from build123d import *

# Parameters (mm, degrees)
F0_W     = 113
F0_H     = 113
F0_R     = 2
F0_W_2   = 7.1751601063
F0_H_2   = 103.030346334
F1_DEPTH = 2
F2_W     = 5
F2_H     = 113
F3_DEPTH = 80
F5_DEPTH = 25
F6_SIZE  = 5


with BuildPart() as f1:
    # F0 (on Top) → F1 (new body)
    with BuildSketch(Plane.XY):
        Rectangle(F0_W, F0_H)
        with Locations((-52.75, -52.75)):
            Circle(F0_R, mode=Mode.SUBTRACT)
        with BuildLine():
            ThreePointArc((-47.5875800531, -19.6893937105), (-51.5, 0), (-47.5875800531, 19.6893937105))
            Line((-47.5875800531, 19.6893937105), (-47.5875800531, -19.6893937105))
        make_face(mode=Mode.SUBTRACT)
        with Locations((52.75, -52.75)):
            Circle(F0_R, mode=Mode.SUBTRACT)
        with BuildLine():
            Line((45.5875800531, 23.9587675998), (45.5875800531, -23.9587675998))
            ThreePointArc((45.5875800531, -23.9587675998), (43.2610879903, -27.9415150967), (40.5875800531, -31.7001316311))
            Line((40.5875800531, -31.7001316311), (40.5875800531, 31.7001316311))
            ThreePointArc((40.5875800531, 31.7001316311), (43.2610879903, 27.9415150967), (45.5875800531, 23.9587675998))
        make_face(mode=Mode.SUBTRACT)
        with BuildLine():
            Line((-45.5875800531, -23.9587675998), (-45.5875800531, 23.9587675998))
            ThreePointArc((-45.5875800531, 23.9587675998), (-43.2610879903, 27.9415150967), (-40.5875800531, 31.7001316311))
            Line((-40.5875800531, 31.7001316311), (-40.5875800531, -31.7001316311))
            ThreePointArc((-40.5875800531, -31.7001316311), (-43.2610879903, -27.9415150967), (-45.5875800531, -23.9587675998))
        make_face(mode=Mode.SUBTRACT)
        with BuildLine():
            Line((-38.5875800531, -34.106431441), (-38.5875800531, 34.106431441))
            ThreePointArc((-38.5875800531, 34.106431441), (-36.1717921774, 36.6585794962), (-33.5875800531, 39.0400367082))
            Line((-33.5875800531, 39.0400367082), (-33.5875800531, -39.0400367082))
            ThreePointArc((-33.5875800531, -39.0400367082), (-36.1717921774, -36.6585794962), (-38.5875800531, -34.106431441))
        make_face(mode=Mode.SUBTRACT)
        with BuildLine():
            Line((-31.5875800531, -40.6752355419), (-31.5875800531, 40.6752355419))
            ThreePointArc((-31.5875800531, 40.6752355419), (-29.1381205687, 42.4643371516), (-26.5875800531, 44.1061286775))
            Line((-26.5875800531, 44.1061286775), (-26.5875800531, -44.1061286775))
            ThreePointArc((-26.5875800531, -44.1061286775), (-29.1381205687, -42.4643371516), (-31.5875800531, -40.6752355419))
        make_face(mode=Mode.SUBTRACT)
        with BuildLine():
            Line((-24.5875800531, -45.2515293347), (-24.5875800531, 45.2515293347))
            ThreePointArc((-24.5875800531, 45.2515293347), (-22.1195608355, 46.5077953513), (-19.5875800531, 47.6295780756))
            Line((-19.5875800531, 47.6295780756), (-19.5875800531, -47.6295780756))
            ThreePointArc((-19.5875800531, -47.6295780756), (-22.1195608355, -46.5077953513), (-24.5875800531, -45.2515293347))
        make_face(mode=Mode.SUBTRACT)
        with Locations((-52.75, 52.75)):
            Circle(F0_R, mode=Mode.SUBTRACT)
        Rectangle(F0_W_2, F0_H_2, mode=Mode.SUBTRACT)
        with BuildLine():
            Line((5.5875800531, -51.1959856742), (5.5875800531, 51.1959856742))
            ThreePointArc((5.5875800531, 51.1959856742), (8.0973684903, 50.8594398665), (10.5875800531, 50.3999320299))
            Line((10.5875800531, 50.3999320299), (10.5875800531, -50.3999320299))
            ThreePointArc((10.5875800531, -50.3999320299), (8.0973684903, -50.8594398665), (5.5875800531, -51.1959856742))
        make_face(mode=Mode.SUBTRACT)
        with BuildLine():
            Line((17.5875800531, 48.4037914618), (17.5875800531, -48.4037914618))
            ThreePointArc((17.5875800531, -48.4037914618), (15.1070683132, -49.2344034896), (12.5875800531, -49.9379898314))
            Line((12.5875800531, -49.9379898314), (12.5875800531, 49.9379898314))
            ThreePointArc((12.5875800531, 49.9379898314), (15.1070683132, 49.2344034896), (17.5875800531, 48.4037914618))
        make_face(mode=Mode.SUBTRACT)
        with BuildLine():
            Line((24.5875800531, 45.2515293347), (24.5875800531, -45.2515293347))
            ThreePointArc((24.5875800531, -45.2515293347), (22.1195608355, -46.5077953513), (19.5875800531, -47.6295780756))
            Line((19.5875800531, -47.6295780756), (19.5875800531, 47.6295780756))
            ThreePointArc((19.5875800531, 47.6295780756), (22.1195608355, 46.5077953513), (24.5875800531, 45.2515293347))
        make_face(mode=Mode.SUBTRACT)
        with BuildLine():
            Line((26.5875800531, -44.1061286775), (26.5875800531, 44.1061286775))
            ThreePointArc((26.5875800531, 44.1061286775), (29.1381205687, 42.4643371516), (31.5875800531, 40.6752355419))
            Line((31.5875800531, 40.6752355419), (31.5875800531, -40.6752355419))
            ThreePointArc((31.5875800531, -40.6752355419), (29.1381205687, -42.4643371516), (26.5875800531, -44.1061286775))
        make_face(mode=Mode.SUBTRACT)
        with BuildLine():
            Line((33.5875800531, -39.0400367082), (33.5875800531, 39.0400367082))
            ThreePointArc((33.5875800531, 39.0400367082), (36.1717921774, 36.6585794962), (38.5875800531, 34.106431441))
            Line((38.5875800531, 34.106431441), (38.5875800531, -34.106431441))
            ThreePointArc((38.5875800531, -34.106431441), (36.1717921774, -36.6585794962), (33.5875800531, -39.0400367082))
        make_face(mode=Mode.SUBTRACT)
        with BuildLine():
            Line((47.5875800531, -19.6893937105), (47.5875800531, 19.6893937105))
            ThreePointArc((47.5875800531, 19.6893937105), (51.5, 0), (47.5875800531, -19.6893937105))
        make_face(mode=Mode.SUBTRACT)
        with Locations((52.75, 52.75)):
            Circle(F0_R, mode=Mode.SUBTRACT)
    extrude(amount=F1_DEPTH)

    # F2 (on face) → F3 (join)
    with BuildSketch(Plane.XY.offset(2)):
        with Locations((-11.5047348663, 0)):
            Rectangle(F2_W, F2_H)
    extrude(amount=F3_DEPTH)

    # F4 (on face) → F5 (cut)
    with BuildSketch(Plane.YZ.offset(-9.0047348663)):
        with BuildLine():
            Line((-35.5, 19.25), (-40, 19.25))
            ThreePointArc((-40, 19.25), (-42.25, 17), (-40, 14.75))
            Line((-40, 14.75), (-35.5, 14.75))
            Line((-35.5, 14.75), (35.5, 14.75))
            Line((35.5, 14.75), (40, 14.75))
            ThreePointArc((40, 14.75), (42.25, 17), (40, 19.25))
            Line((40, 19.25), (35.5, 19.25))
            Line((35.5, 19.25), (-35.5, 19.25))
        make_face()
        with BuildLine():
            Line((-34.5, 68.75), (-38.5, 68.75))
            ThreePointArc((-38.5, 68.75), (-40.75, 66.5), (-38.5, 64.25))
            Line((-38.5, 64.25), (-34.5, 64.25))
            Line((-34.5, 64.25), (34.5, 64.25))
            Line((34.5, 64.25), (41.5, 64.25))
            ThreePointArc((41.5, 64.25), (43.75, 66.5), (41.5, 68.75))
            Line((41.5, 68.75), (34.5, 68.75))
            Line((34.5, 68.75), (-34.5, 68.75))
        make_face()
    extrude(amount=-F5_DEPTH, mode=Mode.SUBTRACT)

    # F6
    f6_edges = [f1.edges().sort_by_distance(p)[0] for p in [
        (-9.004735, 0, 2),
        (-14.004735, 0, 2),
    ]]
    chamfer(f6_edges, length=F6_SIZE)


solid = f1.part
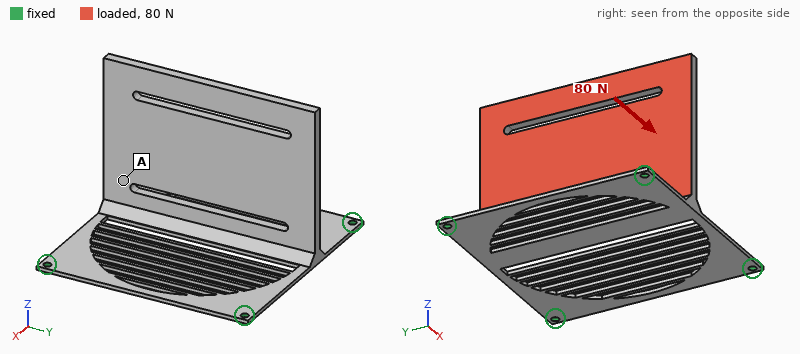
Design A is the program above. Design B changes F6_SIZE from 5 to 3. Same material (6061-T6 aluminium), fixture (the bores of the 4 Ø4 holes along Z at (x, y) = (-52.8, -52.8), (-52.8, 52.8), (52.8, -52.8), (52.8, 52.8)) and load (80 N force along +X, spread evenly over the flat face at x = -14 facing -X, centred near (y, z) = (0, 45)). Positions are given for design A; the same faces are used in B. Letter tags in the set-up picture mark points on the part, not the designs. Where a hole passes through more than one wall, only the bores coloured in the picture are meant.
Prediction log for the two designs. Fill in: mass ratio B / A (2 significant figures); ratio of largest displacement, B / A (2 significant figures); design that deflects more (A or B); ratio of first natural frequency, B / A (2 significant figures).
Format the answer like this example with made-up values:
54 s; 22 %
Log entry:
0.97; 1.1; B; 0.95
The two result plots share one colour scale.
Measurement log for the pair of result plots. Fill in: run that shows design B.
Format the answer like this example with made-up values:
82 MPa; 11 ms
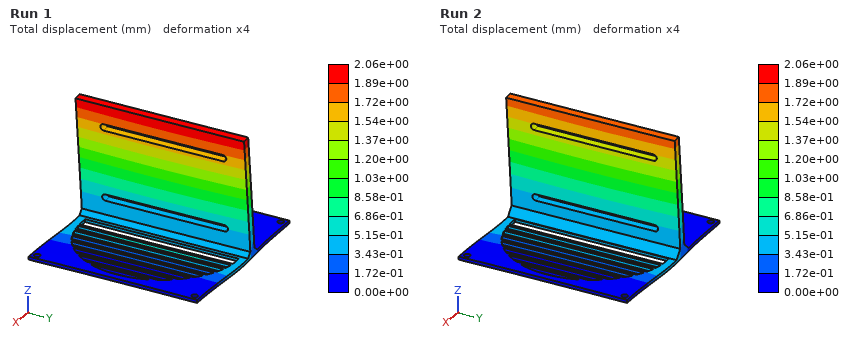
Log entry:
Run 1
